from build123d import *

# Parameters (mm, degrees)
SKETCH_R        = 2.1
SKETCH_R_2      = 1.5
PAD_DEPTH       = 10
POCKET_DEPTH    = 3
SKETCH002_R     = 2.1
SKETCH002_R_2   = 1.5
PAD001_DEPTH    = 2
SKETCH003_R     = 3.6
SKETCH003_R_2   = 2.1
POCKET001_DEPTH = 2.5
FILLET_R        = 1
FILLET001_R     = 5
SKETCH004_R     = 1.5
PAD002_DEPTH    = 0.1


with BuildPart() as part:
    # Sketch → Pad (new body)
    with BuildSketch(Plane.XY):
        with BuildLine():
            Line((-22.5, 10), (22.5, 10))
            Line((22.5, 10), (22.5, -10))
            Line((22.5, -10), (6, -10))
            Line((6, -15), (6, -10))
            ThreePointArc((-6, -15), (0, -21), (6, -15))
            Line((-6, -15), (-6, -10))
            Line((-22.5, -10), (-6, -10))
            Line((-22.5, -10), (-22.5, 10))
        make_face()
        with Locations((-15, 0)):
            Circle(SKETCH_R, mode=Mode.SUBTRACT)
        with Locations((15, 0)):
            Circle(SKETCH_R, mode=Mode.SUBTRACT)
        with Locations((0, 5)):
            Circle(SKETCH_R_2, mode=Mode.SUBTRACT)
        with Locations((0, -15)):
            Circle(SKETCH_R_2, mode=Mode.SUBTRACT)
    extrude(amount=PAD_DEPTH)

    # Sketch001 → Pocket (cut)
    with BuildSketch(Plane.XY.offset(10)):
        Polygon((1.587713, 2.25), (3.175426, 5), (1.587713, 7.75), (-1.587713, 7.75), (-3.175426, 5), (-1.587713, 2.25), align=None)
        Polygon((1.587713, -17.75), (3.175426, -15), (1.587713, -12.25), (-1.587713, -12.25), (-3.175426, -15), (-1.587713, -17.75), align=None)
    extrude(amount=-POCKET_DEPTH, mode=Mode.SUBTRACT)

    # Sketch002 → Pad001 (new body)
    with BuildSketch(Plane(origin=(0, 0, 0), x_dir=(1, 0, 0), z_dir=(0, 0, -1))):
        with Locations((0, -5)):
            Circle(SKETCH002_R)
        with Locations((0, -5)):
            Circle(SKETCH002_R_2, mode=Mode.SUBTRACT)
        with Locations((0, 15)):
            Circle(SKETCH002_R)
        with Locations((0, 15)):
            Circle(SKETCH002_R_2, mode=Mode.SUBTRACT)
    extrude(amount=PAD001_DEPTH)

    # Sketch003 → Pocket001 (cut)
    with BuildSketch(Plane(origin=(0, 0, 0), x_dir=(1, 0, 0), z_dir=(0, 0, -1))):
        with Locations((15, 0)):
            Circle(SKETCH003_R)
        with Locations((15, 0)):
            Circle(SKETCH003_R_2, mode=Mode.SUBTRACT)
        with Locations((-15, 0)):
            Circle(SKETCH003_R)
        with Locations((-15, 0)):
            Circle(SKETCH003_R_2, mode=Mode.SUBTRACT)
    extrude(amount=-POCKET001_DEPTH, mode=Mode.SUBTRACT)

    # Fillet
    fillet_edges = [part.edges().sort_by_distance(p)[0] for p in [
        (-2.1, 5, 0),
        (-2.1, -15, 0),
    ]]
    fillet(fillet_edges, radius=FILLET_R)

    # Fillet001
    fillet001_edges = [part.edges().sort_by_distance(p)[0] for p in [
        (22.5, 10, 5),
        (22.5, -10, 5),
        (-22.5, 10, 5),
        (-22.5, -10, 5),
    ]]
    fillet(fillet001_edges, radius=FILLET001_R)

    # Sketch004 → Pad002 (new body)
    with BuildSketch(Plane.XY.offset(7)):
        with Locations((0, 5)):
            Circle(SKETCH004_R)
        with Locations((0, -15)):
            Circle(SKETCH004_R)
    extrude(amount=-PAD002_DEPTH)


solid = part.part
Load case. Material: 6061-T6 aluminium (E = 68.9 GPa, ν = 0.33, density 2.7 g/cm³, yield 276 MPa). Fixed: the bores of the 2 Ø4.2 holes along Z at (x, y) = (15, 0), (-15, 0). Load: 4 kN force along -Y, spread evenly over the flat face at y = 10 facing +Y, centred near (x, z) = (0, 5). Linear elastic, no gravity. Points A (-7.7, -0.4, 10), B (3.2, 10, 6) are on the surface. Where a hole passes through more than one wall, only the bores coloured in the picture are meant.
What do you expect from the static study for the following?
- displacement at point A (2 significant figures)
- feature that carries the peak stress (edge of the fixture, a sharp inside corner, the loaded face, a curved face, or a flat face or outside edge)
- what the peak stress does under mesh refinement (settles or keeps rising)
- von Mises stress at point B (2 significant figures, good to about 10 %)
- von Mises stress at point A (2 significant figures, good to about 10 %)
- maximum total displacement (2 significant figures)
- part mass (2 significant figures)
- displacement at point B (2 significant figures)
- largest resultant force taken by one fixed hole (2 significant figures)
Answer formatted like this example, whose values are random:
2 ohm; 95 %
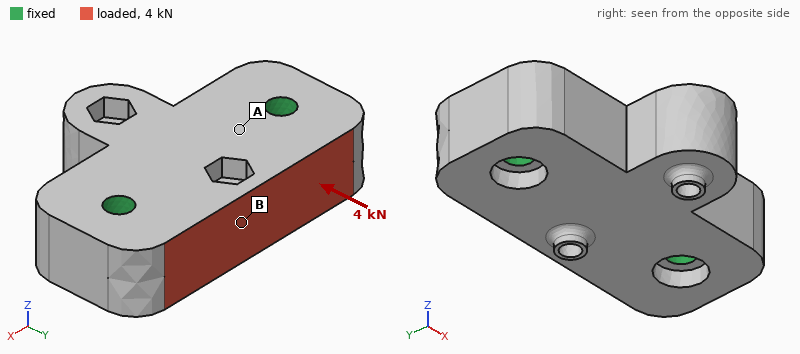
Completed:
2.6 µm; edge of the fixture; keeps rising; 18 MPa; 8.5 MPa; 7.4 µm; 25 g; 5.8 µm; 2.0 kN
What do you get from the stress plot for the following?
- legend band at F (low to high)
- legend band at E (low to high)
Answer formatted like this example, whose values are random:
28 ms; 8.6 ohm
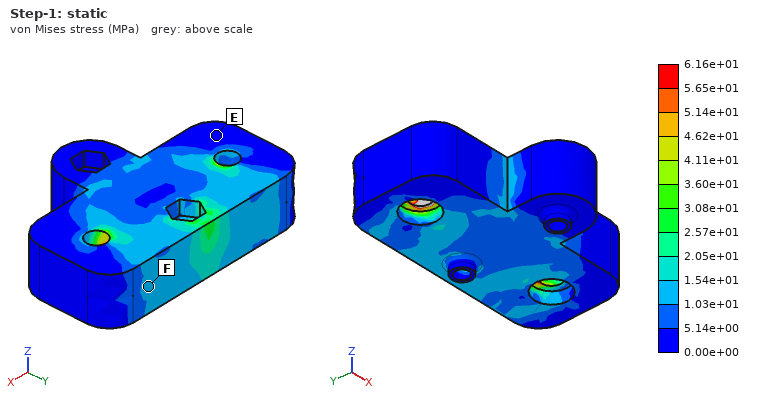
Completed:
1.03e+01 to 1.54e+01 MPa; 0.00e+00 to 5.14e+00 MPa
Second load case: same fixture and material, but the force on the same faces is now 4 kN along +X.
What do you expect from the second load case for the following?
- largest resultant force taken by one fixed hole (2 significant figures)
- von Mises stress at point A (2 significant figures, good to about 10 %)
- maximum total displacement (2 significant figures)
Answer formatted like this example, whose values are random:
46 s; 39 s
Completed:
2.3 kN; 12 MPa; 6.4 µm
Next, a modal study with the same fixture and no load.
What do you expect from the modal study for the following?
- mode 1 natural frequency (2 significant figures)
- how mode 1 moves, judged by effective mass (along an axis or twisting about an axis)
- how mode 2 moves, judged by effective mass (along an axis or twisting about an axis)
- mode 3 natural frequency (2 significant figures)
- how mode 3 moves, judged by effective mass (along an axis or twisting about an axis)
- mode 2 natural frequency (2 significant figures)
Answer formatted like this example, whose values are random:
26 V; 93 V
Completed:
15 kHz; along Z; along Z; 33 kHz; along Y; 28 kHz
